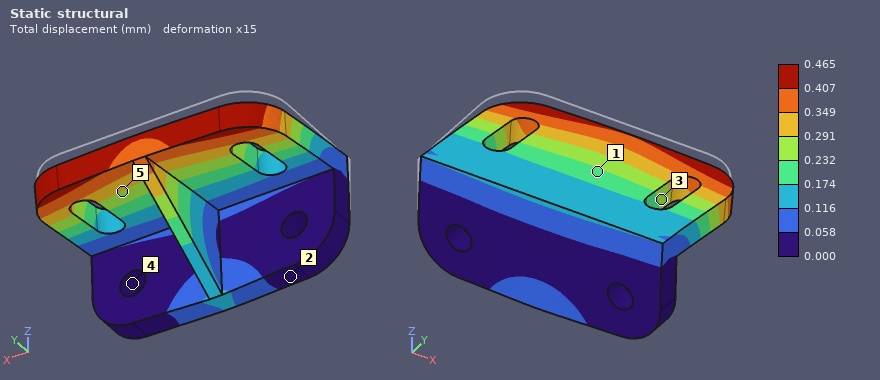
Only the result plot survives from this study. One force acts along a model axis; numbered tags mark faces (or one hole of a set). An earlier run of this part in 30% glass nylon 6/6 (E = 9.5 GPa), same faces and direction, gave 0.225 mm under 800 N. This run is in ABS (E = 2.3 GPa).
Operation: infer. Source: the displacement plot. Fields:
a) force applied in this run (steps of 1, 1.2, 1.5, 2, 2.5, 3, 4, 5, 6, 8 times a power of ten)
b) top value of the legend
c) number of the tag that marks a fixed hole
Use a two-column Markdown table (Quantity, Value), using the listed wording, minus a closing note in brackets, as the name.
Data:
| Quantity | Value |
|---|---|
| force applied in this run | 400 N |
| top value of the legend | 0.465 mm |
| number of the tag that marks a fixed hole | 4 |
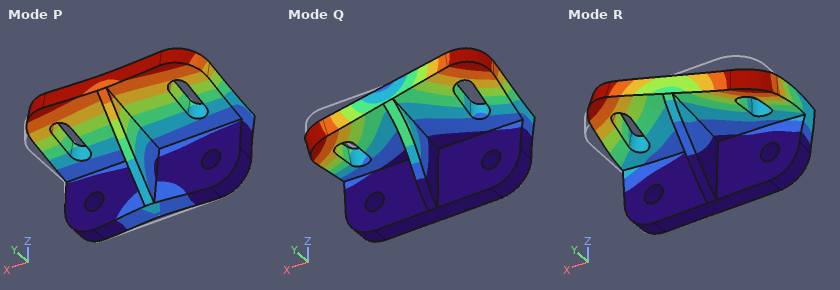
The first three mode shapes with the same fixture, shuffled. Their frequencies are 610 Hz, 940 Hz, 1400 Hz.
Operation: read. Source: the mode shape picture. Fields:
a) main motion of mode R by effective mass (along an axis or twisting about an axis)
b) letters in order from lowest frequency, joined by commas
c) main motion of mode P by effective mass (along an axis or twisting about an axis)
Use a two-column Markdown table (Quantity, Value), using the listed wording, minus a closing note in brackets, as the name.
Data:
| Quantity | Value |
|---|---|
| main motion of mode R by effective mass | along X |
| letters in order from lowest frequency, joined by commas | P, Q, R |
| main motion of mode P by effective mass | along Z |
